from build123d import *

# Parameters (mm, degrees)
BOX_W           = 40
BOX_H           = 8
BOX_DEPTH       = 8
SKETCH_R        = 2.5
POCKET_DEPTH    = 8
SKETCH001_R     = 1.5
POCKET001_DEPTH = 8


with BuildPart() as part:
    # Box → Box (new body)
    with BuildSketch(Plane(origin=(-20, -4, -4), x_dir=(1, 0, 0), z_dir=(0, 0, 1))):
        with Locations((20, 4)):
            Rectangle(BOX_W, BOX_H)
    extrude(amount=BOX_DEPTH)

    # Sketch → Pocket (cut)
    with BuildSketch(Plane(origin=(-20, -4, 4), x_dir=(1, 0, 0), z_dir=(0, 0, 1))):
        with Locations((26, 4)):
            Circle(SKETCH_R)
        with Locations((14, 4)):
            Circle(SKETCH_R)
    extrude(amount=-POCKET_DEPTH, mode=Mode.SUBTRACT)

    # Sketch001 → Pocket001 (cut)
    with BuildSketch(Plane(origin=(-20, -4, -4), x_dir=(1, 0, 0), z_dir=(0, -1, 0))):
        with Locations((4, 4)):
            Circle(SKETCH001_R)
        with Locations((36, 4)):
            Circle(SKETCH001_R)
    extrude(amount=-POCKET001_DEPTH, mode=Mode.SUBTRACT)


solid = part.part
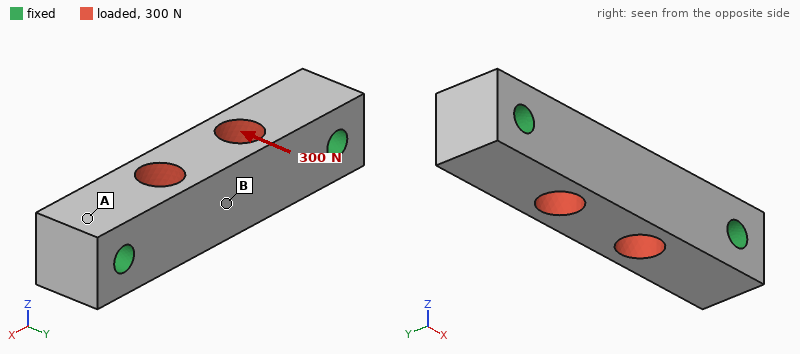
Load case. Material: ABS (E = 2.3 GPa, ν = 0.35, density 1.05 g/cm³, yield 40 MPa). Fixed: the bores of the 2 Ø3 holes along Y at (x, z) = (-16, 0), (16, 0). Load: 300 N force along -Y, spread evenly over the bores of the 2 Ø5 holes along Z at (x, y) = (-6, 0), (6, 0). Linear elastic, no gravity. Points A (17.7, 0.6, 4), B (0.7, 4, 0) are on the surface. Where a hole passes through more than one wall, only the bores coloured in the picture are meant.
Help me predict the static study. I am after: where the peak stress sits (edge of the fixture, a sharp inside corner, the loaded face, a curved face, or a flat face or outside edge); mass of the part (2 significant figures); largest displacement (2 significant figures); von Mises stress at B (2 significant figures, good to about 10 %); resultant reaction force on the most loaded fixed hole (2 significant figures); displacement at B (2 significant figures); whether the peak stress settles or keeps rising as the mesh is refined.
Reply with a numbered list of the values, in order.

1. edge of the fixture
2. 2.2 g
3. 0.13 mm
4. 7.0 MPa
5. 150 N
6. 0.12 mm
7. keeps rising
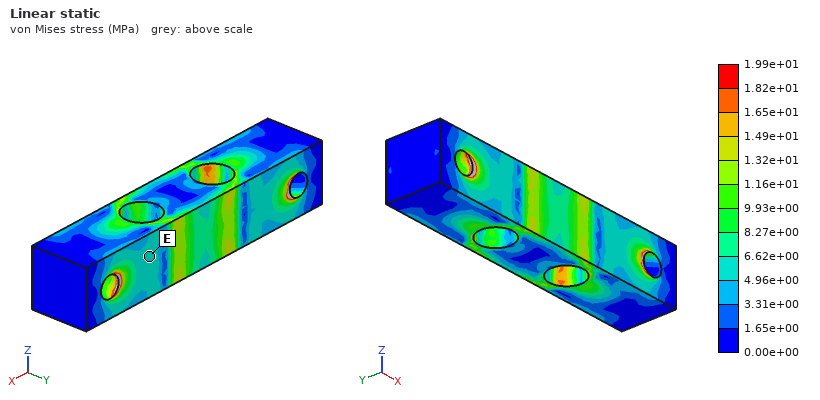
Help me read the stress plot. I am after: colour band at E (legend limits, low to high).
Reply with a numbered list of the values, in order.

1. 4.96e+00 to 6.62e+00 MPa
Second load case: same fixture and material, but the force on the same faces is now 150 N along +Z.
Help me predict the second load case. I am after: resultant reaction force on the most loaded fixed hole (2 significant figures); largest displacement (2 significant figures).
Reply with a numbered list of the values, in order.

1. 75 N
2. 59 µm
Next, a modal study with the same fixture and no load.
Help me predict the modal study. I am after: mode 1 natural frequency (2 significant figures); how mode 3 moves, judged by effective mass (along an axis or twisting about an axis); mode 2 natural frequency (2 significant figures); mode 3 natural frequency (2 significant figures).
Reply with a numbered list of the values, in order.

1. 7600 Hz
2. twisting about X
3. 7900 Hz
4. 12 kHz
